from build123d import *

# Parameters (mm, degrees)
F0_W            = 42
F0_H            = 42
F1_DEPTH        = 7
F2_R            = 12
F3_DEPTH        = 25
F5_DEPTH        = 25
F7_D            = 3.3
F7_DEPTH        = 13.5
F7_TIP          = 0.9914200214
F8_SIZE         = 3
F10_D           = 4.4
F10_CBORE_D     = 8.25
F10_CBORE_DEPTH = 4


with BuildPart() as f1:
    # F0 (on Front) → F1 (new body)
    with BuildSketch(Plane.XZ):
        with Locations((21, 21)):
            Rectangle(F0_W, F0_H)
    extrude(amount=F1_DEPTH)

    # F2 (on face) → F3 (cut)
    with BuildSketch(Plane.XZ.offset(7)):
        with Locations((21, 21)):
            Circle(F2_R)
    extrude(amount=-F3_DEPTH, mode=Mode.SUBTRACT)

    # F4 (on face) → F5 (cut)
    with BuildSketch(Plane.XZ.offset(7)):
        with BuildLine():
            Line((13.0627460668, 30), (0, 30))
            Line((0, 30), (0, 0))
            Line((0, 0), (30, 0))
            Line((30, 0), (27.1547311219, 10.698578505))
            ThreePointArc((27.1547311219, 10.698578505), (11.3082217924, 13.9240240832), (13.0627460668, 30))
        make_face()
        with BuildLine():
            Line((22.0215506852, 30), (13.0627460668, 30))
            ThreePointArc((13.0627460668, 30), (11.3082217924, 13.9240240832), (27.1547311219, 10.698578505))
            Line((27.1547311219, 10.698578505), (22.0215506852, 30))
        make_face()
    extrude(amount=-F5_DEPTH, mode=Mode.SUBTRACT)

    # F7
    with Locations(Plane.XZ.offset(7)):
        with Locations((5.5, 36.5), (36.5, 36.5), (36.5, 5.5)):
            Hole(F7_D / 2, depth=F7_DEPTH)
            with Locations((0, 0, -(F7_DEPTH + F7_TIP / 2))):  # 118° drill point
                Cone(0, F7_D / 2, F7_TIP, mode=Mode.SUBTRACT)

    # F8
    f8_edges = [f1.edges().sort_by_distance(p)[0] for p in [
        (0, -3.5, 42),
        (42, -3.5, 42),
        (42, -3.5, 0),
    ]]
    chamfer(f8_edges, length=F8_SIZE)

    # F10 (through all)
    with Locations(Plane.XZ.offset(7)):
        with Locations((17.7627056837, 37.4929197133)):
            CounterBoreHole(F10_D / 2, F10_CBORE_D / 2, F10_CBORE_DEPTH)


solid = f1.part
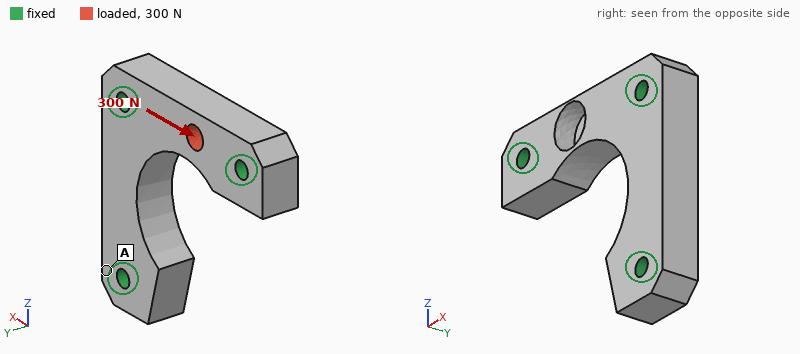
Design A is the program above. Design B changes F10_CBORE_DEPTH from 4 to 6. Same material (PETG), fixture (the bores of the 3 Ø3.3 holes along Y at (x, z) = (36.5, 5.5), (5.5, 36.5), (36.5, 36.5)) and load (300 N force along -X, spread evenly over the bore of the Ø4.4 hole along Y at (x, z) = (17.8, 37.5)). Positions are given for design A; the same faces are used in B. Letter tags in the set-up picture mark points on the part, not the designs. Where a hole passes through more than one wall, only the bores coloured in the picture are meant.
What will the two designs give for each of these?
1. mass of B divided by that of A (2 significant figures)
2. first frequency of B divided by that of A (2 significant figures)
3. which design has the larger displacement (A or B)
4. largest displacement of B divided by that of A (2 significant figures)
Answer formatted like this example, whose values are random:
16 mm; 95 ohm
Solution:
0.99; 0.97; B; 2.2
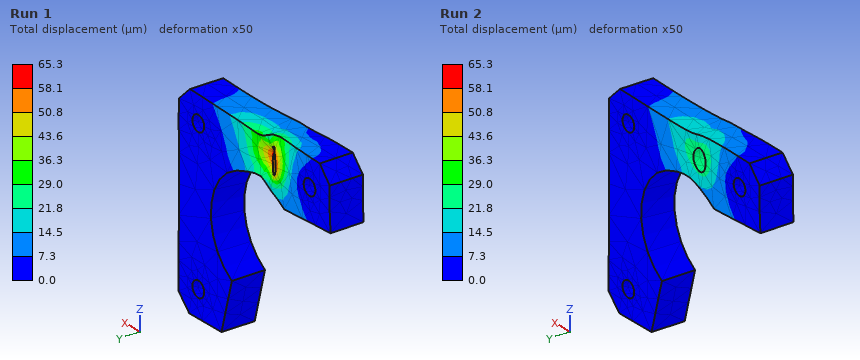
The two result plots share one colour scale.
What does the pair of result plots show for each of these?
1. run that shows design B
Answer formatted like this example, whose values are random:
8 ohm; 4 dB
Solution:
Run 1
